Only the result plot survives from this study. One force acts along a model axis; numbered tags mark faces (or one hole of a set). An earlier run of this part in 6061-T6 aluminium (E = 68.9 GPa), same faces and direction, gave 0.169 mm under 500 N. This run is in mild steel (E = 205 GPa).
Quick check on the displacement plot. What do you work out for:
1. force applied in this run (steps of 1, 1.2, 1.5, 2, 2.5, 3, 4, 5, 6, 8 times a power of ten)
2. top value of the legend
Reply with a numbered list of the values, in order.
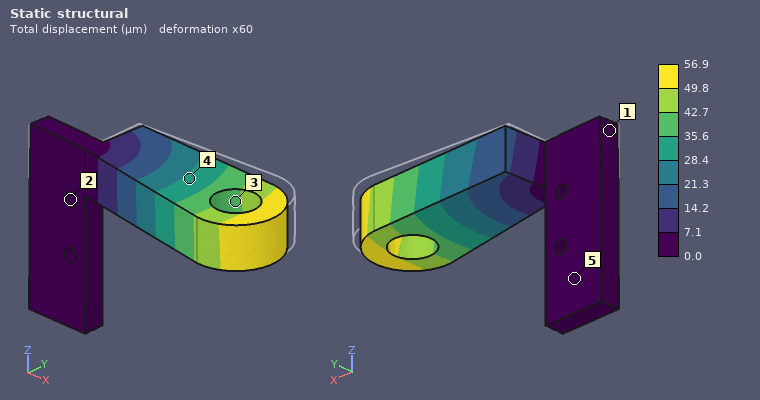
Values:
1. 500 N
2. 56.9 µm
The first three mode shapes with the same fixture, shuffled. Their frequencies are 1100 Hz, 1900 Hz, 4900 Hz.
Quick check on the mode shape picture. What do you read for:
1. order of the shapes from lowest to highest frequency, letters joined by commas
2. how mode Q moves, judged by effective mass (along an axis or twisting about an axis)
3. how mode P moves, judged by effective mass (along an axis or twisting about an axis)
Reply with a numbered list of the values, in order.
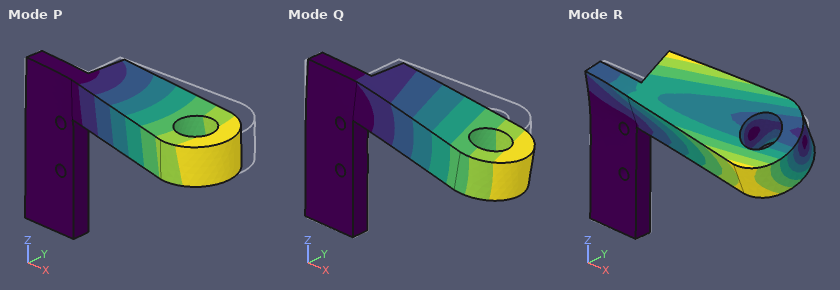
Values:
1. P, Q, R
2. along Z
3. along Y
